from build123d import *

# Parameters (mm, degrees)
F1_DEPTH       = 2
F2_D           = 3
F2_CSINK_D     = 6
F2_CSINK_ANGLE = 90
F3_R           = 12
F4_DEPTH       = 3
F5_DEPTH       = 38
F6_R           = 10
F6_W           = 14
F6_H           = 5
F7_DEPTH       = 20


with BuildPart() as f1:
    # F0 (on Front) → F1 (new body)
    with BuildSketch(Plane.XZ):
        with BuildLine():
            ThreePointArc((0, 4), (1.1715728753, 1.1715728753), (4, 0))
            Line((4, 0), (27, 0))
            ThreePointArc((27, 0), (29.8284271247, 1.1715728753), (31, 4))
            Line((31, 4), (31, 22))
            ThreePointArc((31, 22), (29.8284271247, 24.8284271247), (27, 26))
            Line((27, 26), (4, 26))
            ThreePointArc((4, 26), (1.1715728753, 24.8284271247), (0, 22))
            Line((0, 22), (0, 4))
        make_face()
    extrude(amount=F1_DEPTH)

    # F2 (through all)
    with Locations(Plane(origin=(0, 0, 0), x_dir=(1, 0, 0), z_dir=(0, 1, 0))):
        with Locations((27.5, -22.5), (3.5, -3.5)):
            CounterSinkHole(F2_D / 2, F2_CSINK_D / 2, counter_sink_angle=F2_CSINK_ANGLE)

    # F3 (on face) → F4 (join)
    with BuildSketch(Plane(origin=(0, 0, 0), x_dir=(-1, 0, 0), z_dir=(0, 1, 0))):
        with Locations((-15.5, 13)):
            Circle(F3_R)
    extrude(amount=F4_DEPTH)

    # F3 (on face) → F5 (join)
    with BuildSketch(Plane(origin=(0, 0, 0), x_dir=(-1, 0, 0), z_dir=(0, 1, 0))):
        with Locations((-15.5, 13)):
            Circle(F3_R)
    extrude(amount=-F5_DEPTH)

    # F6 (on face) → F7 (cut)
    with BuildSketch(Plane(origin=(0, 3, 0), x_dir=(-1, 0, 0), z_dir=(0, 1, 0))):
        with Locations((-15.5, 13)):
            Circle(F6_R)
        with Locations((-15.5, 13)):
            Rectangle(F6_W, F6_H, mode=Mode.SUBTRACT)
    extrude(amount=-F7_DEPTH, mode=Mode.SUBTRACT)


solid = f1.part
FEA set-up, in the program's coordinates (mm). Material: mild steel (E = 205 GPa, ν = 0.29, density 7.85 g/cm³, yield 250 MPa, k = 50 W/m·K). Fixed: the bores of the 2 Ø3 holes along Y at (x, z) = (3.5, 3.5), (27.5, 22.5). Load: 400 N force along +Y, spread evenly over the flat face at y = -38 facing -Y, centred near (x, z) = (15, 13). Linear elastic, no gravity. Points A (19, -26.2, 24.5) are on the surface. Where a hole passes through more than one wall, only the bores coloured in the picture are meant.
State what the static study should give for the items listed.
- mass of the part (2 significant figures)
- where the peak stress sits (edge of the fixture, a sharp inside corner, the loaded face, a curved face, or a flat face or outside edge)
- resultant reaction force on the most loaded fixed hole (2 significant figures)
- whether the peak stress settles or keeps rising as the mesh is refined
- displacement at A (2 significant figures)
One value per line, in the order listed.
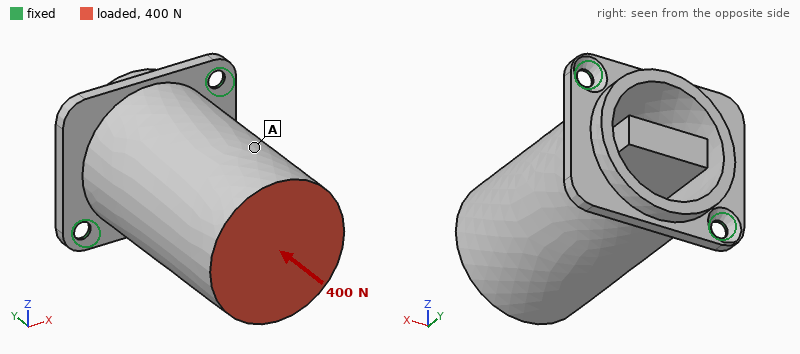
110 g
edge of the fixture
200 N
keeps rising
3.6 µm
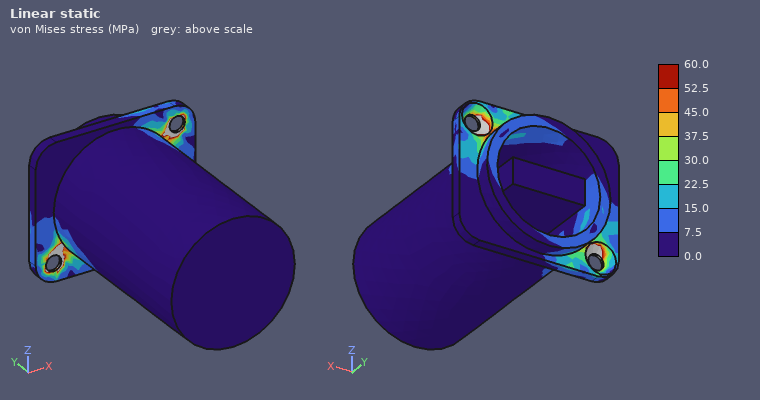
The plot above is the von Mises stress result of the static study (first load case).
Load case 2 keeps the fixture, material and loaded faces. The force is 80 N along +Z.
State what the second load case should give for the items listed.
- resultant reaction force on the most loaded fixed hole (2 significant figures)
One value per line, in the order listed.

78 N
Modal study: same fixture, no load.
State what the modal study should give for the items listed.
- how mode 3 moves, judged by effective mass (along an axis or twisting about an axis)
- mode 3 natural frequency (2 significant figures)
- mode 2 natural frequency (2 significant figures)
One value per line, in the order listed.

along Y
5000 Hz
2800 Hz
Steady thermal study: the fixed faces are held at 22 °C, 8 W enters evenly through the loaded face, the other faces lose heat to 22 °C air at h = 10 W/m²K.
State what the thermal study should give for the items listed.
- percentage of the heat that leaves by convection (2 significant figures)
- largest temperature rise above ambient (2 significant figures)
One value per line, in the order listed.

24 %
44 K
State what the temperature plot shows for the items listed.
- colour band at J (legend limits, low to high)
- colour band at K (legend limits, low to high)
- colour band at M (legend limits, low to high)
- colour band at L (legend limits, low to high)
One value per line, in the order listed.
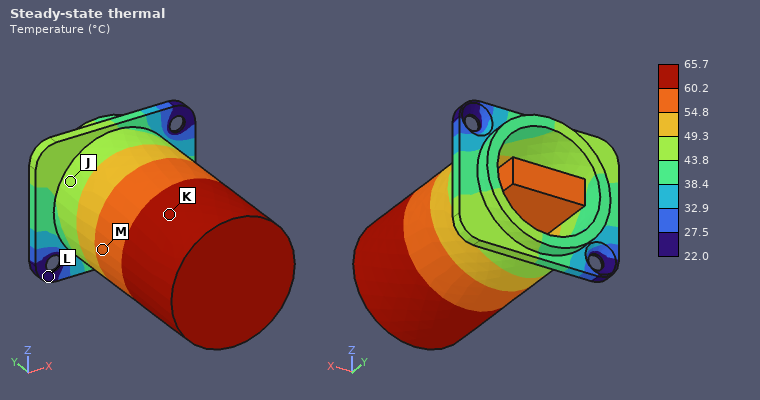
43.8 to 49.3 °C
60.2 to 65.7 °C
54.8 to 60.2 °C
22.0 to 27.5 °C
